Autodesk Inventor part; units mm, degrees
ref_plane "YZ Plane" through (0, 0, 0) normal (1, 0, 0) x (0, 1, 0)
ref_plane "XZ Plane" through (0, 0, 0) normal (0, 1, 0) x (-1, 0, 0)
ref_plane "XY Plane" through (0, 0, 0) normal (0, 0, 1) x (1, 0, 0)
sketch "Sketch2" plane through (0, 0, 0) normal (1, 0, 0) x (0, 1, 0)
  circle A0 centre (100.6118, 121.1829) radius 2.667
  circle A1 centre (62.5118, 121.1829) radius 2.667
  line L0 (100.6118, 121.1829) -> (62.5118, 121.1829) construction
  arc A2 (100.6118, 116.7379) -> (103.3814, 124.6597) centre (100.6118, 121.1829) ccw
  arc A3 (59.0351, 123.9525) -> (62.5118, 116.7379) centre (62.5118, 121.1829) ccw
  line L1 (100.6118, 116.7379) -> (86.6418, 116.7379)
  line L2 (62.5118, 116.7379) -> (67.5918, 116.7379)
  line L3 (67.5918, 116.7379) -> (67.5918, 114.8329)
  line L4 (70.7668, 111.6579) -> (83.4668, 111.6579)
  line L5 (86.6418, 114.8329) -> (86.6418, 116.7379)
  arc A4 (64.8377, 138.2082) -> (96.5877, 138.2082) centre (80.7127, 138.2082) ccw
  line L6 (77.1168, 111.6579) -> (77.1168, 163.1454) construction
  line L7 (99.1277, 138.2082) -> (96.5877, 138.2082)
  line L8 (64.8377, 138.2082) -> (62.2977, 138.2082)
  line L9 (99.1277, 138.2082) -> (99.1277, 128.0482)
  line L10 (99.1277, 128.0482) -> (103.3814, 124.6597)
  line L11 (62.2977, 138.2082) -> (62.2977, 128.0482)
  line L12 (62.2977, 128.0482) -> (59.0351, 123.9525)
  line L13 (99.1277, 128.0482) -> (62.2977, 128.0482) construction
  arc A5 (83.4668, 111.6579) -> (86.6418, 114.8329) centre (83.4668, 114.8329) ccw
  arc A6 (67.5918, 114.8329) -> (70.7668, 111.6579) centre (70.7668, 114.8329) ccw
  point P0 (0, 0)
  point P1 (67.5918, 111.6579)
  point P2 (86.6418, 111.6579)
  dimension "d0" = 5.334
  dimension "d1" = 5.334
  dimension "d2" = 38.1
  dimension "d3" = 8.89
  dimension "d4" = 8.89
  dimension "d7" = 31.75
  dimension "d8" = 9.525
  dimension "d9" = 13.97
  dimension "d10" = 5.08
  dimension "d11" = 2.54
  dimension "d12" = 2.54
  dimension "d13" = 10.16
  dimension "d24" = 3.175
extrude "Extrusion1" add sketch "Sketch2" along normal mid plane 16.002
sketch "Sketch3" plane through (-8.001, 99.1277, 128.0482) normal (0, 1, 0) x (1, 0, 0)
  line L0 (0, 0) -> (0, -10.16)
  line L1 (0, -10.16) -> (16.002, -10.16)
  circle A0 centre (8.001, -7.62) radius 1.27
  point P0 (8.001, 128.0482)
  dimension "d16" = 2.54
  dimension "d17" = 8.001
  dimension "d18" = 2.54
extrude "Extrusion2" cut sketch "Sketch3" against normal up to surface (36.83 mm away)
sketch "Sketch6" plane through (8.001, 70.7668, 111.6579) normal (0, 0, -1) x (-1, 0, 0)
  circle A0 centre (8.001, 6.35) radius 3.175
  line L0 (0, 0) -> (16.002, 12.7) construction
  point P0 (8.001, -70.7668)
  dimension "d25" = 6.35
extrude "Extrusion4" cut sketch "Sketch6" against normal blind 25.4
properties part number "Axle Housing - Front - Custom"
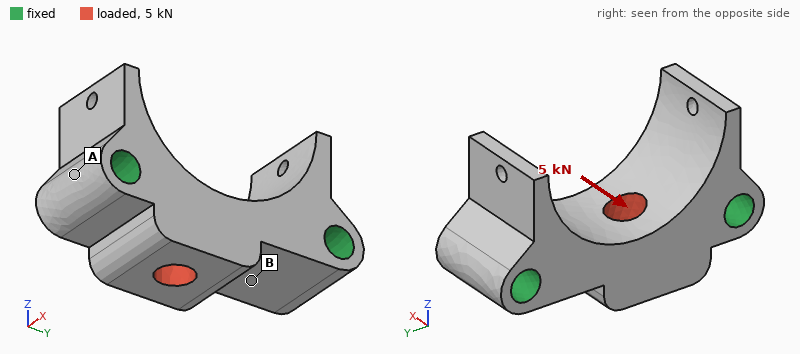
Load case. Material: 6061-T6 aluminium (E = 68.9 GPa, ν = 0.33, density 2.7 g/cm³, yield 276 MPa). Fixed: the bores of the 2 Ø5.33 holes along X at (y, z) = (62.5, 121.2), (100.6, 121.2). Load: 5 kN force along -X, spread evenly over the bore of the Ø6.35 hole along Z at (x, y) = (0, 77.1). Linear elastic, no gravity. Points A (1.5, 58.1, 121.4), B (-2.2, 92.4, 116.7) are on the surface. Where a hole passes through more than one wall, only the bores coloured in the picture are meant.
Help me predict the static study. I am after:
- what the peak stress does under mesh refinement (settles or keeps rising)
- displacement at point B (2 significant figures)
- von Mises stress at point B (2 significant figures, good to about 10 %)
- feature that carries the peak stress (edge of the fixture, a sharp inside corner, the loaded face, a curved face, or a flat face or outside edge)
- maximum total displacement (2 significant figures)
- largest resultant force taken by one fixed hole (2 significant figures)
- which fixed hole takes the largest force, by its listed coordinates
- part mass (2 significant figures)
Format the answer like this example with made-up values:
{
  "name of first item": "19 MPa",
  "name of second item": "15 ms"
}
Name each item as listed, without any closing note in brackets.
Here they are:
{
  "what the peak stress does under mesh refinement": "keeps rising",
  "displacement at point B": "6.4 µm",
  "von Mises stress at point B": "51 MPa",
  "feature that carries the peak stress": "edge of the fixture",
  "maximum total displacement": "26 µm",
  "largest resultant force taken by one fixed hole": "3.3 kN",
  "which fixed hole takes the largest force, by its listed coordinates": "(62.5, 121.2)",
  "part mass": "22 g"
}
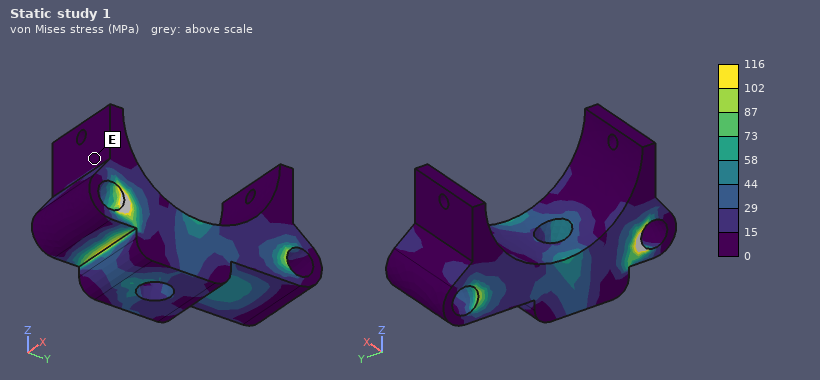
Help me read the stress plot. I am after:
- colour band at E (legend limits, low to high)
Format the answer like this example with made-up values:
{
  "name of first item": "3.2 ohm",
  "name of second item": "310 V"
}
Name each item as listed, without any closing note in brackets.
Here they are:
{
  "colour band at E": "0 to 15 MPa"
}
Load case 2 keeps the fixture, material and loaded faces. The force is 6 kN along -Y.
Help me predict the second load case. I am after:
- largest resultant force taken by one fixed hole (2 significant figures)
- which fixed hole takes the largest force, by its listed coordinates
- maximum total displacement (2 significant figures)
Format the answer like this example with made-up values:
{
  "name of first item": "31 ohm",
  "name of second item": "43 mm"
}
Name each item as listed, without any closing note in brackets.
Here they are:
{
  "largest resultant force taken by one fixed hole": "3.7 kN",
  "which fixed hole takes the largest force, by its listed coordinates": "(62.5, 121.2)",
  "maximum total displacement": "9.5 µm"
}
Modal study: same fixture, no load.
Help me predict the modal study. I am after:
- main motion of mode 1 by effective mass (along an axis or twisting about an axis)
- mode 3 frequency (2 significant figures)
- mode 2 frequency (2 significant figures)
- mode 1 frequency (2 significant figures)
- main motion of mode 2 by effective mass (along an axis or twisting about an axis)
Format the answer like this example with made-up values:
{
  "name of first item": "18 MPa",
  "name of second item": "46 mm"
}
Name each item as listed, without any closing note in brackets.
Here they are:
{
  "main motion of mode 1 by effective mass": "along Z",
  "mode 3 frequency": "32 kHz",
  "mode 2 frequency": "28 kHz",
  "mode 1 frequency": "24 kHz",
  "main motion of mode 2 by effective mass": "along X"
}
